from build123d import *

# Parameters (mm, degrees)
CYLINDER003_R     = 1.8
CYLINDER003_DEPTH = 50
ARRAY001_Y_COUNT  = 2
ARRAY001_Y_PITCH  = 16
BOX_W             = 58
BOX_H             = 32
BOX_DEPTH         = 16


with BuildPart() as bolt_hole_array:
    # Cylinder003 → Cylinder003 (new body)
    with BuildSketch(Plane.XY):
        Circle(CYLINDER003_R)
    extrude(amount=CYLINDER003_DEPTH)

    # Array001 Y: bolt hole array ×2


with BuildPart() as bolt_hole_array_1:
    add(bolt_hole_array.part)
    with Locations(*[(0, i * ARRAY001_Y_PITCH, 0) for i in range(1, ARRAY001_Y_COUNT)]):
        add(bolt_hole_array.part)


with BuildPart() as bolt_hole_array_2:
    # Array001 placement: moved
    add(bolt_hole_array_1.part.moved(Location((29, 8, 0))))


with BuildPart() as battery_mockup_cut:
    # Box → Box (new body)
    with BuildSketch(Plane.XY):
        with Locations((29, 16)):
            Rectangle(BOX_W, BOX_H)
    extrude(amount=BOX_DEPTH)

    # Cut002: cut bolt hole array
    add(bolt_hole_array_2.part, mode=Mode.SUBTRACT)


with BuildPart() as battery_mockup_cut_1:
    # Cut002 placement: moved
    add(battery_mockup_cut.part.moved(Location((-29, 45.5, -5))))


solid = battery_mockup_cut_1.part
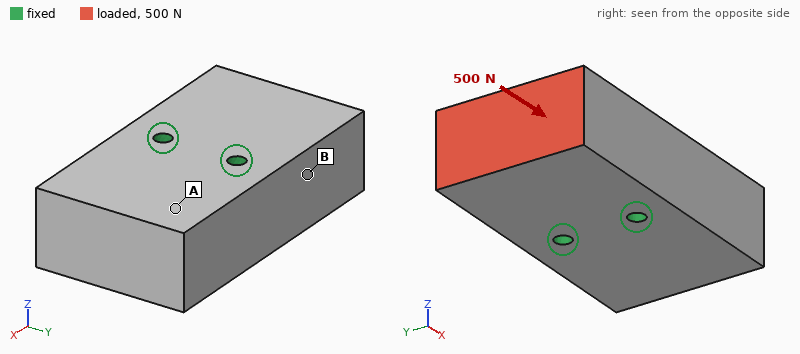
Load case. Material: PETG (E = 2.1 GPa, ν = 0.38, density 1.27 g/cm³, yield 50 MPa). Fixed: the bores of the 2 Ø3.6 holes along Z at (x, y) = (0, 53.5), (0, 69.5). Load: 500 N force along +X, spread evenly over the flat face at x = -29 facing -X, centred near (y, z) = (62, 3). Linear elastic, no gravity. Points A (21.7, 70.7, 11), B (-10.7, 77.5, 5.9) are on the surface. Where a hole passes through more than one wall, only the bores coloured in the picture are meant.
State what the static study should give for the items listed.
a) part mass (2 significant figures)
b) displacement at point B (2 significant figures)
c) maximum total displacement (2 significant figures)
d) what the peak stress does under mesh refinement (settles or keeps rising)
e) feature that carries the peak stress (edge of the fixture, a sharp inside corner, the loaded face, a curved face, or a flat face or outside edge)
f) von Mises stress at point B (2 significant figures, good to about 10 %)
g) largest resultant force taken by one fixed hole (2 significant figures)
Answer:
37 g
7.1 µm
15 µm
keeps rising
edge of the fixture
0.79 MPa
250 N
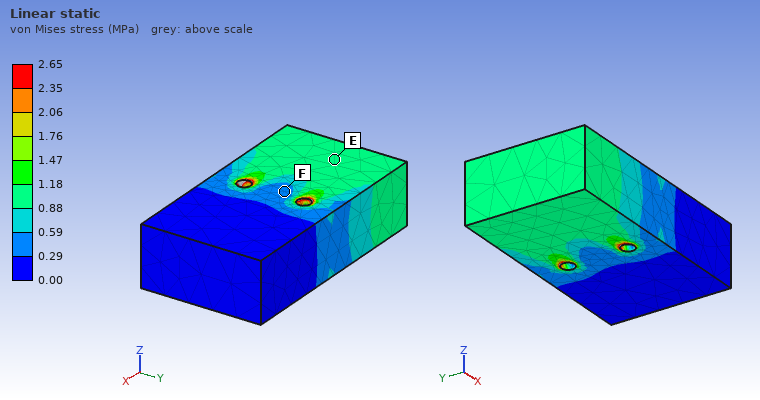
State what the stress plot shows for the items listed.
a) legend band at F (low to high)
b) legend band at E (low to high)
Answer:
0.29 to 0.59 MPa
0.88 to 1.18 MPa
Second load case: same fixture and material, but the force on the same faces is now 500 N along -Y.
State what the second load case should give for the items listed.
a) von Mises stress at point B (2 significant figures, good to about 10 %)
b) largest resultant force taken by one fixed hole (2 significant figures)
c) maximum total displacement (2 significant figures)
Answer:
2.9 MPa
830 N
0.13 mm
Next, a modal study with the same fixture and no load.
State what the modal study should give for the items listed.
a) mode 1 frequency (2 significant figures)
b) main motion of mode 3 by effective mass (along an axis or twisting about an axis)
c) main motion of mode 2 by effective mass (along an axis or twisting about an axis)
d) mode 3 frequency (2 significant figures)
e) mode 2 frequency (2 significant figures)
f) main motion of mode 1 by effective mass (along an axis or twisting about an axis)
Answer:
2800 Hz
twisting about Z
along Z
3600 Hz
3400 Hz
twisting about Y
